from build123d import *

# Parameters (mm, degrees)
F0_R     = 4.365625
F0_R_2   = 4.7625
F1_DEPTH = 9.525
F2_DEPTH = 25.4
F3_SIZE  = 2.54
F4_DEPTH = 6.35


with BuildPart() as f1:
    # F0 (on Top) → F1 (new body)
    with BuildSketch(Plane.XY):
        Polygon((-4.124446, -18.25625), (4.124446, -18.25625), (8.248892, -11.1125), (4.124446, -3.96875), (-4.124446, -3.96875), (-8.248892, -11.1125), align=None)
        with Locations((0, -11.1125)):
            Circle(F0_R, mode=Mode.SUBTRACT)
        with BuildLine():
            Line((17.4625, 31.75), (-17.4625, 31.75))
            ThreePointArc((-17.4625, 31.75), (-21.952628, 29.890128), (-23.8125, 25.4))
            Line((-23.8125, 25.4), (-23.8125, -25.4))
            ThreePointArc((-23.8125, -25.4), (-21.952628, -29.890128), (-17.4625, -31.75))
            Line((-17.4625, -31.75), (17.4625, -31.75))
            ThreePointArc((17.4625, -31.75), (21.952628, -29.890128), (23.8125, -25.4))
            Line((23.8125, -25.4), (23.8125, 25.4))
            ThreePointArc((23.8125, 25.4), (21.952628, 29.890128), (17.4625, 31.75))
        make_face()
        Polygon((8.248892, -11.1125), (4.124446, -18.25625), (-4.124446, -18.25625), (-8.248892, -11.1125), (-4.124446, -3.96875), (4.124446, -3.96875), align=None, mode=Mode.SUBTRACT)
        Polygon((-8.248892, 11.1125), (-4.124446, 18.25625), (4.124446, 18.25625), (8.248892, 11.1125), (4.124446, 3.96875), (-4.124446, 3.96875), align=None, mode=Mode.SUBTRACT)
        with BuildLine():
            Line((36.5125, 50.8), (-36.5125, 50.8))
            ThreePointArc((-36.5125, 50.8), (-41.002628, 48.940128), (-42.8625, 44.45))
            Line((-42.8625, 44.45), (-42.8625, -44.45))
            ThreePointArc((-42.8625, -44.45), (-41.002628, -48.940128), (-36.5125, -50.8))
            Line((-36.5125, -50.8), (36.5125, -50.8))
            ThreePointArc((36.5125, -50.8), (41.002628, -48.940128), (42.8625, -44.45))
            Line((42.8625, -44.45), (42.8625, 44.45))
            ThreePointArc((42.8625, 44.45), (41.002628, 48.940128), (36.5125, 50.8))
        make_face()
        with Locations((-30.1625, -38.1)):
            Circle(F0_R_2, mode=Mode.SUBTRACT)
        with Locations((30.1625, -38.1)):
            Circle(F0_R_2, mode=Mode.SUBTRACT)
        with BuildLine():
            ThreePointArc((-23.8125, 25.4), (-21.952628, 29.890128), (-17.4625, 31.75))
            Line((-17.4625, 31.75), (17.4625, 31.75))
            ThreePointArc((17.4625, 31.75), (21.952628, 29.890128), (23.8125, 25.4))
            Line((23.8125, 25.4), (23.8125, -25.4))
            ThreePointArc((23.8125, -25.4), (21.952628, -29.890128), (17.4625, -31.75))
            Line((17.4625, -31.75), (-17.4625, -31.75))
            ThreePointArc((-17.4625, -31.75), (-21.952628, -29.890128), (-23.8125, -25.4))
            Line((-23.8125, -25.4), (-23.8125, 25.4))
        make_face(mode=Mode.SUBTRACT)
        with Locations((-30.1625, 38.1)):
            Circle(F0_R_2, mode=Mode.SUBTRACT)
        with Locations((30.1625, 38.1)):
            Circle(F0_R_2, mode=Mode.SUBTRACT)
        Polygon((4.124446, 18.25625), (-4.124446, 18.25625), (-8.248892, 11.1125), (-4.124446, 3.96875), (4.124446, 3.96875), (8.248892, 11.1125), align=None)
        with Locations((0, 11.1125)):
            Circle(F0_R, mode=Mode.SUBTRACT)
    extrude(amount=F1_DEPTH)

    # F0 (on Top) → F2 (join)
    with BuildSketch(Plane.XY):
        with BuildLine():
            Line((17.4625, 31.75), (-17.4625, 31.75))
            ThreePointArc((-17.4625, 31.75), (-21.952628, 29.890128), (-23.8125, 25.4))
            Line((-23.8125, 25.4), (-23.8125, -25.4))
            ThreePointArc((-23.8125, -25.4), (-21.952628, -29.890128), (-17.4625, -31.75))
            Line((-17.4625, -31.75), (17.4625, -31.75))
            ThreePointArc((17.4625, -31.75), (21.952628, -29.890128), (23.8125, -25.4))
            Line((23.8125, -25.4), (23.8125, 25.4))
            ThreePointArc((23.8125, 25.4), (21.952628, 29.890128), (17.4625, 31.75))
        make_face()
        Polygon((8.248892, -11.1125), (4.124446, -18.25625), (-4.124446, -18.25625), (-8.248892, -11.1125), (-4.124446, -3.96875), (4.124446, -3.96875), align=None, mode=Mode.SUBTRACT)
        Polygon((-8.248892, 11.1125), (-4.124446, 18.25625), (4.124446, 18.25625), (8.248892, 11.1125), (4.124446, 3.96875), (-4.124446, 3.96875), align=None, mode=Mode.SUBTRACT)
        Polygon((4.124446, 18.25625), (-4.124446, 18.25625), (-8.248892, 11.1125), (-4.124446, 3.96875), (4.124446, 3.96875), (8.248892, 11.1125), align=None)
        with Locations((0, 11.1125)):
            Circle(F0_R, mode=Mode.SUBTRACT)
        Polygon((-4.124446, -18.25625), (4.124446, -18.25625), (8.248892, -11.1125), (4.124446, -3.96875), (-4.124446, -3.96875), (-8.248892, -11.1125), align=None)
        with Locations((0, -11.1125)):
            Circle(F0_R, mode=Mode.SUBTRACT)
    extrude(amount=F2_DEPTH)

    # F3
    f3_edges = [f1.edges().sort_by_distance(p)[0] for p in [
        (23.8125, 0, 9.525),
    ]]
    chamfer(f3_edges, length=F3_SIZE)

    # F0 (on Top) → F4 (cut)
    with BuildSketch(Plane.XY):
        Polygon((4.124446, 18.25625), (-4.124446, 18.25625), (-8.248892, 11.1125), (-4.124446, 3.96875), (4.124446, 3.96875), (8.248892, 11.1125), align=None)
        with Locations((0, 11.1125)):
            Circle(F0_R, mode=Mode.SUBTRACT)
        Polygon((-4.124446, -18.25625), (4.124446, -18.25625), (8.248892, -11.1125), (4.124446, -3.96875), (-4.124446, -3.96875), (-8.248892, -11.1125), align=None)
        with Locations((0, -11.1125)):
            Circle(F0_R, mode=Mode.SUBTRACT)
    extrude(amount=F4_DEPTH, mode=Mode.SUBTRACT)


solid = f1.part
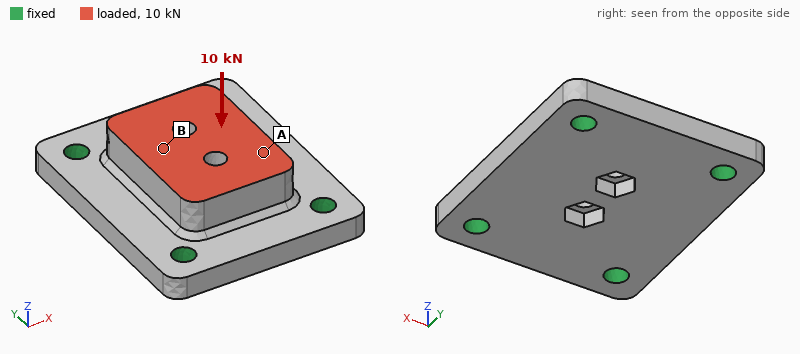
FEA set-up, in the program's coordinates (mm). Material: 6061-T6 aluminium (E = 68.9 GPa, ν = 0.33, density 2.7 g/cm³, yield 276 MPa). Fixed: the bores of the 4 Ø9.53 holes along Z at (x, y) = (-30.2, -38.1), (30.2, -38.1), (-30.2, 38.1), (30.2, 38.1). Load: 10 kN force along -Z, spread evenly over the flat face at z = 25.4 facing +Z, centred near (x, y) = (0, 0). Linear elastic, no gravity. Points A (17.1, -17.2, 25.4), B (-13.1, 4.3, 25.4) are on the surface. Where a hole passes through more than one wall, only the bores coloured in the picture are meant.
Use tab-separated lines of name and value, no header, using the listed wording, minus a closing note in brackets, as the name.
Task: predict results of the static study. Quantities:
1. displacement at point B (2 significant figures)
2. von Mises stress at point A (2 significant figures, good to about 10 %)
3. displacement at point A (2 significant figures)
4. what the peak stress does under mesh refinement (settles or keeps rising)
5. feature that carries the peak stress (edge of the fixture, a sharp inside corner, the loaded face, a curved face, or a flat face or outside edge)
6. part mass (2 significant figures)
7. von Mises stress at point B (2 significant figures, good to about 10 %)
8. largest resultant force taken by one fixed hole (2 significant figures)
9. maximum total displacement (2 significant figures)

displacement at point B	17 µm
von Mises stress at point A	5.1 MPa
displacement at point A	15 µm
what the peak stress does under mesh refinement	keeps rising
feature that carries the peak stress	edge of the fixture
part mass	330 g
von Mises stress at point B	9.8 MPa
largest resultant force taken by one fixed hole	2.9 kN
maximum total displacement	17 µm
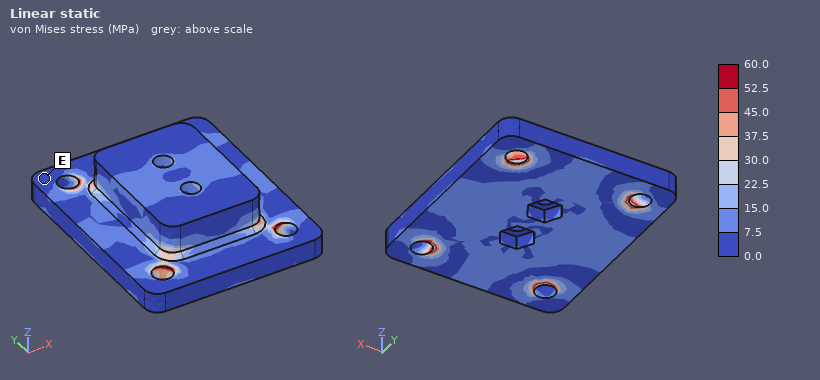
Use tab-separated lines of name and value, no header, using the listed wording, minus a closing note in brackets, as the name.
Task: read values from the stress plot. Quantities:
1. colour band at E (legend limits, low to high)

colour band at E	0.0 to 7.5 MPa
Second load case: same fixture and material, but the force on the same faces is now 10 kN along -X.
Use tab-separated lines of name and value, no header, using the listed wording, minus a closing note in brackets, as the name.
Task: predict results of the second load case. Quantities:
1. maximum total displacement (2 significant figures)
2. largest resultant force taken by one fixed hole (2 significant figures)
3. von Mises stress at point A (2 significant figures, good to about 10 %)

maximum total displacement	18 µm
largest resultant force taken by one fixed hole	3.4 kN
von Mises stress at point A	9.1 MPa
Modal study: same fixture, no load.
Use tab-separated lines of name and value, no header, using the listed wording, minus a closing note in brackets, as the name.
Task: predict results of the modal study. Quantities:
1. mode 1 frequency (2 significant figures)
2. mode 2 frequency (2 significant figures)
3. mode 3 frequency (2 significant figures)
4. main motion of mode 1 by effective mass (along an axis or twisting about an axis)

mode 1 frequency	8300 Hz
mode 2 frequency	11 kHz
mode 3 frequency	13 kHz
main motion of mode 1 by effective mass	along Z
